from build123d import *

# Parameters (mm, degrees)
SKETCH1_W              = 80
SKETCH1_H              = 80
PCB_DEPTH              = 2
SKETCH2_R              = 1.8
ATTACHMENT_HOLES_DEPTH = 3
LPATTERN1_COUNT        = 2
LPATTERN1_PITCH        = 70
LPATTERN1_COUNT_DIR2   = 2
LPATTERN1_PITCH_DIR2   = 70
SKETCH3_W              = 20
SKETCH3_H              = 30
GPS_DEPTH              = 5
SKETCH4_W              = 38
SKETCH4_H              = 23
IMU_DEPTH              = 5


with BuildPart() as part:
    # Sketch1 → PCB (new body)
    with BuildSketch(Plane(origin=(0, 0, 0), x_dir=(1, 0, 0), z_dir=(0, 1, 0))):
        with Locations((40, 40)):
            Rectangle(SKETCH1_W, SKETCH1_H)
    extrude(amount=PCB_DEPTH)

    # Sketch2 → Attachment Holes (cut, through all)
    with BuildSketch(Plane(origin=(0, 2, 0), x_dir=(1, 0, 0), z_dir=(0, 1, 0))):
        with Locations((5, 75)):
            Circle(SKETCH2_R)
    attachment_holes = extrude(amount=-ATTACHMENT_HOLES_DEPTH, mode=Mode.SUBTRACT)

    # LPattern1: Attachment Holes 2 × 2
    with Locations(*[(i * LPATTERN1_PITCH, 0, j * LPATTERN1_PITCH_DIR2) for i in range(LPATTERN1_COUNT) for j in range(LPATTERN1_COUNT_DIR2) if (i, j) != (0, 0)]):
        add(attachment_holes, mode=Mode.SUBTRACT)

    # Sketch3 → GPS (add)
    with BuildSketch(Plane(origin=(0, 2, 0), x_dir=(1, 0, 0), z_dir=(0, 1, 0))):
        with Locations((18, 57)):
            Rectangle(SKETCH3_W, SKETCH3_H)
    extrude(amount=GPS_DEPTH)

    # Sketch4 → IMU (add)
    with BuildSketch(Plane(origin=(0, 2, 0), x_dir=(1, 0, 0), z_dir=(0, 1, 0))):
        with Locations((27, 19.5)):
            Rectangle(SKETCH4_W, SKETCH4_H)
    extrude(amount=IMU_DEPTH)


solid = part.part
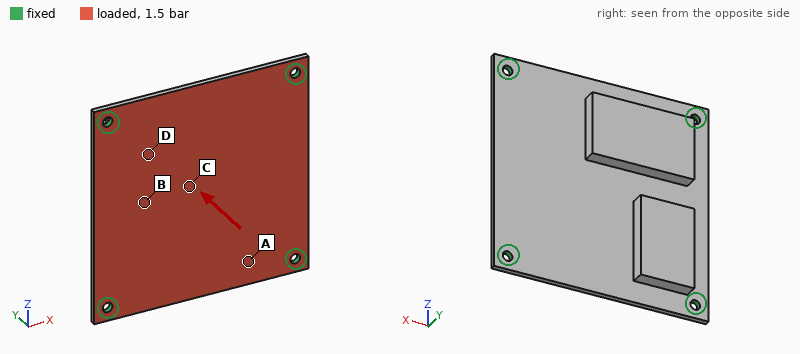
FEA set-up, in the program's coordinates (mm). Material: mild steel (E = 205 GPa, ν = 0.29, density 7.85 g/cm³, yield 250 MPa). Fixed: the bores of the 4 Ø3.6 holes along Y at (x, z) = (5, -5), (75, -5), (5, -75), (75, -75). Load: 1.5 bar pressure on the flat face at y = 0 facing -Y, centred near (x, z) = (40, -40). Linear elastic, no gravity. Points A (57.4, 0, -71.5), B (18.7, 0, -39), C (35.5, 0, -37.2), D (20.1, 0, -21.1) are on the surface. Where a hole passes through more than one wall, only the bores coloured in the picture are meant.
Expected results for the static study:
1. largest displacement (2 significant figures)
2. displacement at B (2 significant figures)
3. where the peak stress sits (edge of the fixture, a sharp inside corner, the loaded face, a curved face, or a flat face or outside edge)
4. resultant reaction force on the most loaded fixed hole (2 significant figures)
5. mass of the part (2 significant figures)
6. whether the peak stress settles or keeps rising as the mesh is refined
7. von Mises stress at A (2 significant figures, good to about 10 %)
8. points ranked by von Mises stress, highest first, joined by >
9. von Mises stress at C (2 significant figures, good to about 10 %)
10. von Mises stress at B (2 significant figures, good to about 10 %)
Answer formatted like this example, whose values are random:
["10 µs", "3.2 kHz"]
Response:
["0.15 mm", "0.10 mm", "edge of the fixture", "280 N", "160 g", "keeps rising", "32 MPa", "B > C > A > D", "62 MPa", "80 MPa"]
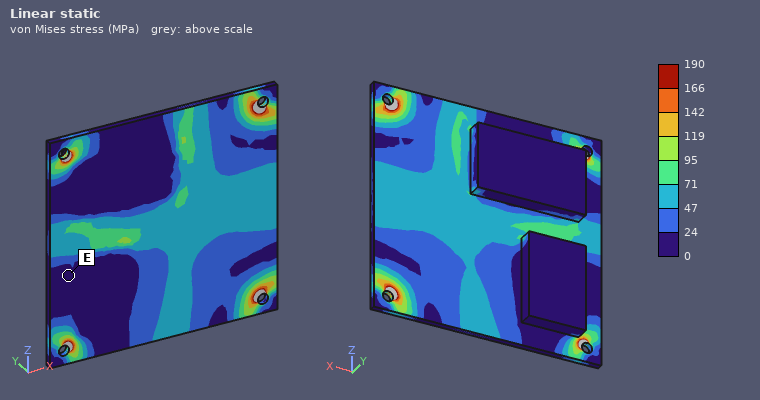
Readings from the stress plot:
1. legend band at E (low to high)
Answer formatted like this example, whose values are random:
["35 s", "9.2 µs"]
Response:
["0 to 24 MPa"]
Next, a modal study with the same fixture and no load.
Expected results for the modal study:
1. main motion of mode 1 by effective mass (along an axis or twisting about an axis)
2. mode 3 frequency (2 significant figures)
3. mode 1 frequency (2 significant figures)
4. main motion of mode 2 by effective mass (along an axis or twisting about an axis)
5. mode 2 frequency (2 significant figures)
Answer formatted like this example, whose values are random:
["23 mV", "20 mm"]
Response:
["along Y", "2900 Hz", "1300 Hz", "twisting about Z", "2600 Hz"]
